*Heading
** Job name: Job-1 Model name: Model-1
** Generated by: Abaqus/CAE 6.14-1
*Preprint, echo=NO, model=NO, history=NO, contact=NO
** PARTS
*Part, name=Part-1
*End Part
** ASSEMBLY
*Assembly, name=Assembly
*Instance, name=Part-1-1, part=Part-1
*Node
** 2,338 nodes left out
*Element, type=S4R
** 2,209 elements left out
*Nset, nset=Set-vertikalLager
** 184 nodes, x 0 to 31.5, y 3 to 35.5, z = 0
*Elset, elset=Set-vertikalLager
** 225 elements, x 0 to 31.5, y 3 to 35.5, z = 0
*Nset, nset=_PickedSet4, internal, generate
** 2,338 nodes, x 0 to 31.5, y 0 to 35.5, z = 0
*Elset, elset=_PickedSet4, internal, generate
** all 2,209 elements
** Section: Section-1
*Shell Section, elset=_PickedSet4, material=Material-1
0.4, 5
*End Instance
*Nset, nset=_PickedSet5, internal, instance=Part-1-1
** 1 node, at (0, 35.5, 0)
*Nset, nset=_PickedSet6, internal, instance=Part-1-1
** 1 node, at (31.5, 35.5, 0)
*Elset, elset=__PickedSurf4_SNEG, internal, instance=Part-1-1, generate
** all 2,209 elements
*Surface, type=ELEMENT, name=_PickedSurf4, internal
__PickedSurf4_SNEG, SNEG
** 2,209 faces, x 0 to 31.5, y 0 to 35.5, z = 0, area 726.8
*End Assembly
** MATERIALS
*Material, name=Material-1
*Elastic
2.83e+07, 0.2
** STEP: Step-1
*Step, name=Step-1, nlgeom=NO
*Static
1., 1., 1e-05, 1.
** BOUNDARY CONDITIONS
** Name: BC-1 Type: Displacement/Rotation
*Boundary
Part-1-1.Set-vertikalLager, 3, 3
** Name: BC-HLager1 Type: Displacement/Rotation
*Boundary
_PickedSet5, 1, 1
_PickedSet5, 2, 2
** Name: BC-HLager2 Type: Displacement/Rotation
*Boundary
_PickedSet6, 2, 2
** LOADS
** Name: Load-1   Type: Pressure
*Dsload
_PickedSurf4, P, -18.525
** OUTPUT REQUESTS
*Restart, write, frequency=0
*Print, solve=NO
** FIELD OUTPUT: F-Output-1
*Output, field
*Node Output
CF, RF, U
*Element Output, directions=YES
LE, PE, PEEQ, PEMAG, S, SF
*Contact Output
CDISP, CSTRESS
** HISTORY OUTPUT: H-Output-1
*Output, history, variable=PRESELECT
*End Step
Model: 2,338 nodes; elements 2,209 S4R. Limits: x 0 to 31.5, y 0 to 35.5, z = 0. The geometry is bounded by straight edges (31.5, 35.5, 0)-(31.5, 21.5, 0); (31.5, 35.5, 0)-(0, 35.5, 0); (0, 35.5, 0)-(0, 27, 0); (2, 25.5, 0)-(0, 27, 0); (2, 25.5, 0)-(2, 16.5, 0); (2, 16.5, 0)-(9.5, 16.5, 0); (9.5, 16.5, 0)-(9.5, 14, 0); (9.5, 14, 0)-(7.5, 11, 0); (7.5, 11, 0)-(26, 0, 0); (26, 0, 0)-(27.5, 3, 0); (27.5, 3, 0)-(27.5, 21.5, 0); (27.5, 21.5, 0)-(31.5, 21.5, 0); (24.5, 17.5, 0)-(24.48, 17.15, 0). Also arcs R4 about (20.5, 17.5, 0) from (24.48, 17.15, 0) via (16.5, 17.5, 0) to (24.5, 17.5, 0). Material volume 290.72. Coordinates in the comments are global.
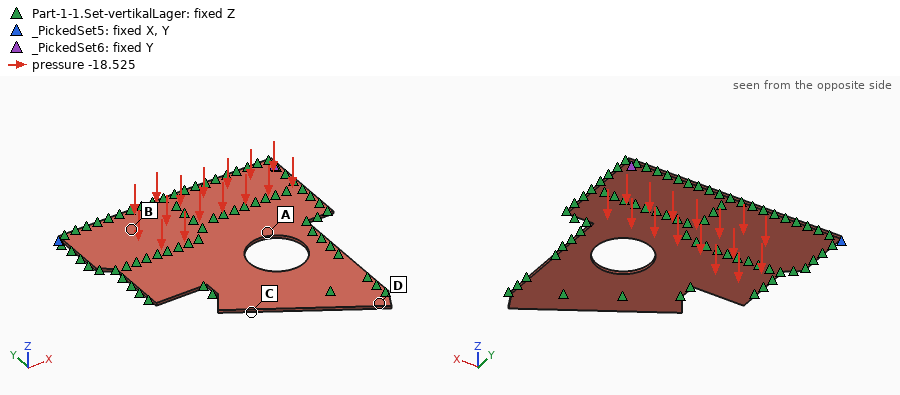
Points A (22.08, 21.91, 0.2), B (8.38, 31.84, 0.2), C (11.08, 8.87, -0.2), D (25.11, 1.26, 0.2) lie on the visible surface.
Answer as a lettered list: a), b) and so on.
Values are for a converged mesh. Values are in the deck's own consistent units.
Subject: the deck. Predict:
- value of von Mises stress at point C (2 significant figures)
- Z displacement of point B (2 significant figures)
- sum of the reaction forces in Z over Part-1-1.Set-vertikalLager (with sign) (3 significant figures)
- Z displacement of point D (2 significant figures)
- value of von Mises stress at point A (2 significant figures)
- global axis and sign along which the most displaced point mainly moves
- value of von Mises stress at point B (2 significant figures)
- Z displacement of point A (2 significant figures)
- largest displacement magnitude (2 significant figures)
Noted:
a) 1100
b) -0.0052
c) 13500
d) -0.0044
e) 5200
f) -Z
g) 3500
h) -0.013
i) 0.019
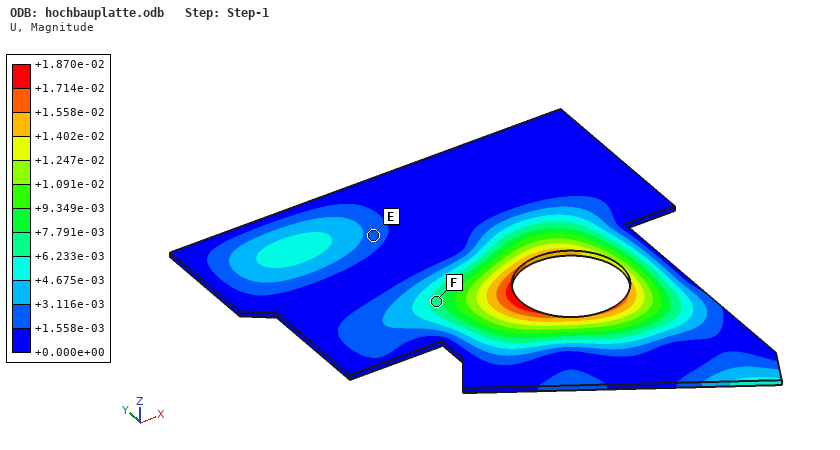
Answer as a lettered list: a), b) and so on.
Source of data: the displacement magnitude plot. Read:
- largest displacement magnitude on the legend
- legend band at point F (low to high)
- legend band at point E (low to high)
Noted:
a) +1.870e-02
b) +6.233e-03 to +7.791e-03
c) +1.558e-03 to +3.116e-03
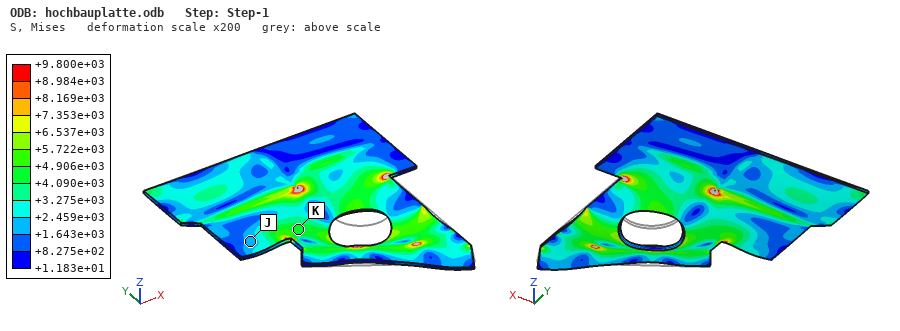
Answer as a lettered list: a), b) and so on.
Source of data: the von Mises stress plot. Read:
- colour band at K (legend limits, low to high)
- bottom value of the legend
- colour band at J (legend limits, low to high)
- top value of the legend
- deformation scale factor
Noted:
a) +4.090e+03 to +4.906e+03
b) +1.183e+01
c) +1.643e+03 to +2.459e+03
d) +9.800e+03
e) 200
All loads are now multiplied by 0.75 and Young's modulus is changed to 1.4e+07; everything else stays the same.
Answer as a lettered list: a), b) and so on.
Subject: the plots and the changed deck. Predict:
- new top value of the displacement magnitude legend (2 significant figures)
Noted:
a) 0.028
